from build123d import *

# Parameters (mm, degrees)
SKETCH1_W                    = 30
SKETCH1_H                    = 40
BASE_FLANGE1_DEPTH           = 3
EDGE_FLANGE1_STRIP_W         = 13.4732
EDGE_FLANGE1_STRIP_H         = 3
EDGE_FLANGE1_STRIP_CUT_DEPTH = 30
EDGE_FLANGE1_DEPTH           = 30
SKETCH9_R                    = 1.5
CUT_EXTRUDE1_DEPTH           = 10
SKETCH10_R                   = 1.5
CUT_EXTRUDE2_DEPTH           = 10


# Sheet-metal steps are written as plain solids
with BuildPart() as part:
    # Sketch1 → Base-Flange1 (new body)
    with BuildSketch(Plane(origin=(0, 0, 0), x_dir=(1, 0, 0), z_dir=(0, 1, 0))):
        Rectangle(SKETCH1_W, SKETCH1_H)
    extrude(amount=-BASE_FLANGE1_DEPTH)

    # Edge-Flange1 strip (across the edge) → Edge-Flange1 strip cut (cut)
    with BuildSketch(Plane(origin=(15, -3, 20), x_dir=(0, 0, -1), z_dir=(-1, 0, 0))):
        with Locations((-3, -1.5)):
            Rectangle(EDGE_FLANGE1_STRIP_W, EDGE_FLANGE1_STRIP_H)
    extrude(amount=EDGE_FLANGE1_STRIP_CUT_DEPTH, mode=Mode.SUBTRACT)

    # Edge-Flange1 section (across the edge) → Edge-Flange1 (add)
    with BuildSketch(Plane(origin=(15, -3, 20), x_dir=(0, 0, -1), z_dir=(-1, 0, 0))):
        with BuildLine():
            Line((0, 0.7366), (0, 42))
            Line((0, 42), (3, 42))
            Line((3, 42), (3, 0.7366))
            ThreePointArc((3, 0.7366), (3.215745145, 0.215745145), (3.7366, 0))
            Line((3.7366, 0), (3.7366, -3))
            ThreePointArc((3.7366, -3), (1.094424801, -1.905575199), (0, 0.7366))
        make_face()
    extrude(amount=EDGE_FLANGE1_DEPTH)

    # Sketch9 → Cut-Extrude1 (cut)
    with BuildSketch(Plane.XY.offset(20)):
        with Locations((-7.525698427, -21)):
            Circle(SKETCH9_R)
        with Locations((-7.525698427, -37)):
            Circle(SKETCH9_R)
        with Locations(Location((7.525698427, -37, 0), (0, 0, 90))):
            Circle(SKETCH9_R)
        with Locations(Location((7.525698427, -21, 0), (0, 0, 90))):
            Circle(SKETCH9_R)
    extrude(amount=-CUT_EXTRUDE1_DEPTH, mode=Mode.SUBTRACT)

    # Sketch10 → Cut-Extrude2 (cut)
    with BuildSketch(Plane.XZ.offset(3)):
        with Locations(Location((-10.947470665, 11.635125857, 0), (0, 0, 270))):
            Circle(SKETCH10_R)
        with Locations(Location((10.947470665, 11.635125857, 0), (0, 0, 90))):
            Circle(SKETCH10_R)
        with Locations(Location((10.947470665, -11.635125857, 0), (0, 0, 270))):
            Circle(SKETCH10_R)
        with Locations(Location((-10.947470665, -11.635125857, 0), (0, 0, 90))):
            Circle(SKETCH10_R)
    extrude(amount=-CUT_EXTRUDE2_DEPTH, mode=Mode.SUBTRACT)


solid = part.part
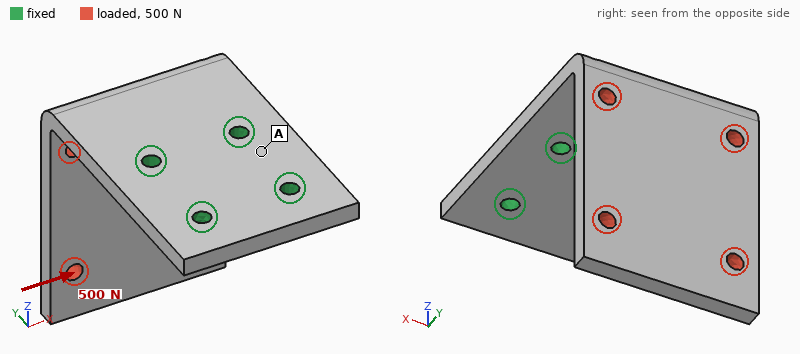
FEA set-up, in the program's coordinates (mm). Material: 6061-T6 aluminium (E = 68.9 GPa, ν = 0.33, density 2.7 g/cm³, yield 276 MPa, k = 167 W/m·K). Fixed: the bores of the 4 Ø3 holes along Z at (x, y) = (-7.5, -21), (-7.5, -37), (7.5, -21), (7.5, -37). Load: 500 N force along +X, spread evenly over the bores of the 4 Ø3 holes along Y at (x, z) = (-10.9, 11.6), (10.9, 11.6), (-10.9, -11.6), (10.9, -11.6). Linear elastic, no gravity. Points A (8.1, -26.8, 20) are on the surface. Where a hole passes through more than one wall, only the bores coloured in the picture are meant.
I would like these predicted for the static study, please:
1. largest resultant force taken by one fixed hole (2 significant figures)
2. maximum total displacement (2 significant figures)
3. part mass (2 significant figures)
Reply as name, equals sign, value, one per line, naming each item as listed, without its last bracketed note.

largest resultant force taken by one fixed hole = 720 N
maximum total displacement = 0.62 mm
part mass = 19 g
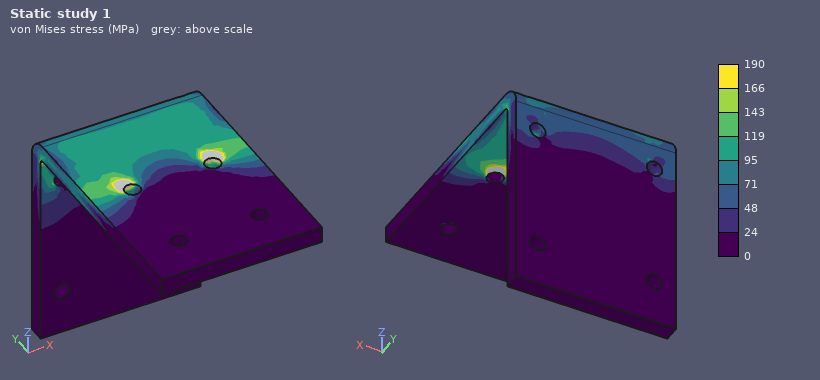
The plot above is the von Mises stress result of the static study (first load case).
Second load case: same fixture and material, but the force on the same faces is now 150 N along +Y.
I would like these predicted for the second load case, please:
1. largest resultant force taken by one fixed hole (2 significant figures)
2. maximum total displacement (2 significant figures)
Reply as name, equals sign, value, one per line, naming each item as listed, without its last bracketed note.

largest resultant force taken by one fixed hole = 69 N
maximum total displacement = 0.63 mm
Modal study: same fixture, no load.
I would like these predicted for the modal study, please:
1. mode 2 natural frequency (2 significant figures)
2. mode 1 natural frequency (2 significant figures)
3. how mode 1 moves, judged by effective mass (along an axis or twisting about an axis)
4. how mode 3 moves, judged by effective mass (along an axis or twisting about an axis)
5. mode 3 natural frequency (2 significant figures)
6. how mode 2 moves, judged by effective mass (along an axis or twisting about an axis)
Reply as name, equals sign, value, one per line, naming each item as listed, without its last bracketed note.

mode 2 natural frequency = 1700 Hz
mode 1 natural frequency = 940 Hz
how mode 1 moves, judged by effective mass = along Y
how mode 3 moves, judged by effective mass = along Z
mode 3 natural frequency = 3200 Hz
how mode 2 moves, judged by effective mass = along X
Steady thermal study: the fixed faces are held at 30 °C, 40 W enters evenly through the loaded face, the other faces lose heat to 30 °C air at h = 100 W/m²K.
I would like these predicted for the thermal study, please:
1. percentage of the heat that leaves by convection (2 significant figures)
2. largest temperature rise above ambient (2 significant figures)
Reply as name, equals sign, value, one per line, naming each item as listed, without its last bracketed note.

percentage of the heat that leaves by convection = 39 %
largest temperature rise above ambient = 68 K
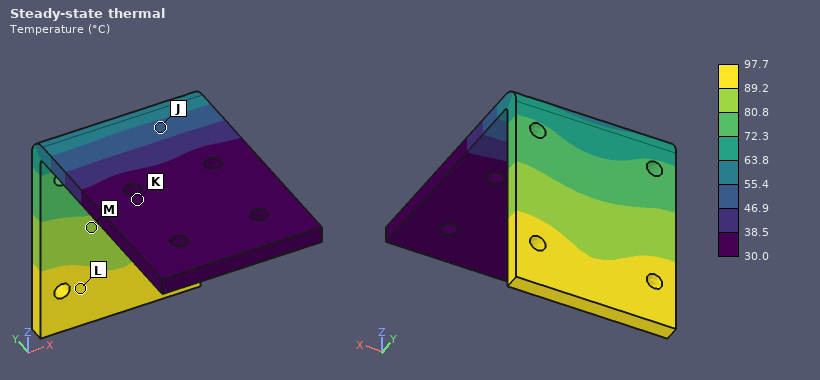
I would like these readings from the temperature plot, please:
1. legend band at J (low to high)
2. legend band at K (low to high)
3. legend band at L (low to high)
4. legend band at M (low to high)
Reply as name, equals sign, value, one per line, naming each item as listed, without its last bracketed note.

legend band at J = 46.9 to 55.4 °C
legend band at K = 30.0 to 38.5 °C
legend band at L = 89.2 to 97.7 °C
legend band at M = 80.8 to 89.2 °C
